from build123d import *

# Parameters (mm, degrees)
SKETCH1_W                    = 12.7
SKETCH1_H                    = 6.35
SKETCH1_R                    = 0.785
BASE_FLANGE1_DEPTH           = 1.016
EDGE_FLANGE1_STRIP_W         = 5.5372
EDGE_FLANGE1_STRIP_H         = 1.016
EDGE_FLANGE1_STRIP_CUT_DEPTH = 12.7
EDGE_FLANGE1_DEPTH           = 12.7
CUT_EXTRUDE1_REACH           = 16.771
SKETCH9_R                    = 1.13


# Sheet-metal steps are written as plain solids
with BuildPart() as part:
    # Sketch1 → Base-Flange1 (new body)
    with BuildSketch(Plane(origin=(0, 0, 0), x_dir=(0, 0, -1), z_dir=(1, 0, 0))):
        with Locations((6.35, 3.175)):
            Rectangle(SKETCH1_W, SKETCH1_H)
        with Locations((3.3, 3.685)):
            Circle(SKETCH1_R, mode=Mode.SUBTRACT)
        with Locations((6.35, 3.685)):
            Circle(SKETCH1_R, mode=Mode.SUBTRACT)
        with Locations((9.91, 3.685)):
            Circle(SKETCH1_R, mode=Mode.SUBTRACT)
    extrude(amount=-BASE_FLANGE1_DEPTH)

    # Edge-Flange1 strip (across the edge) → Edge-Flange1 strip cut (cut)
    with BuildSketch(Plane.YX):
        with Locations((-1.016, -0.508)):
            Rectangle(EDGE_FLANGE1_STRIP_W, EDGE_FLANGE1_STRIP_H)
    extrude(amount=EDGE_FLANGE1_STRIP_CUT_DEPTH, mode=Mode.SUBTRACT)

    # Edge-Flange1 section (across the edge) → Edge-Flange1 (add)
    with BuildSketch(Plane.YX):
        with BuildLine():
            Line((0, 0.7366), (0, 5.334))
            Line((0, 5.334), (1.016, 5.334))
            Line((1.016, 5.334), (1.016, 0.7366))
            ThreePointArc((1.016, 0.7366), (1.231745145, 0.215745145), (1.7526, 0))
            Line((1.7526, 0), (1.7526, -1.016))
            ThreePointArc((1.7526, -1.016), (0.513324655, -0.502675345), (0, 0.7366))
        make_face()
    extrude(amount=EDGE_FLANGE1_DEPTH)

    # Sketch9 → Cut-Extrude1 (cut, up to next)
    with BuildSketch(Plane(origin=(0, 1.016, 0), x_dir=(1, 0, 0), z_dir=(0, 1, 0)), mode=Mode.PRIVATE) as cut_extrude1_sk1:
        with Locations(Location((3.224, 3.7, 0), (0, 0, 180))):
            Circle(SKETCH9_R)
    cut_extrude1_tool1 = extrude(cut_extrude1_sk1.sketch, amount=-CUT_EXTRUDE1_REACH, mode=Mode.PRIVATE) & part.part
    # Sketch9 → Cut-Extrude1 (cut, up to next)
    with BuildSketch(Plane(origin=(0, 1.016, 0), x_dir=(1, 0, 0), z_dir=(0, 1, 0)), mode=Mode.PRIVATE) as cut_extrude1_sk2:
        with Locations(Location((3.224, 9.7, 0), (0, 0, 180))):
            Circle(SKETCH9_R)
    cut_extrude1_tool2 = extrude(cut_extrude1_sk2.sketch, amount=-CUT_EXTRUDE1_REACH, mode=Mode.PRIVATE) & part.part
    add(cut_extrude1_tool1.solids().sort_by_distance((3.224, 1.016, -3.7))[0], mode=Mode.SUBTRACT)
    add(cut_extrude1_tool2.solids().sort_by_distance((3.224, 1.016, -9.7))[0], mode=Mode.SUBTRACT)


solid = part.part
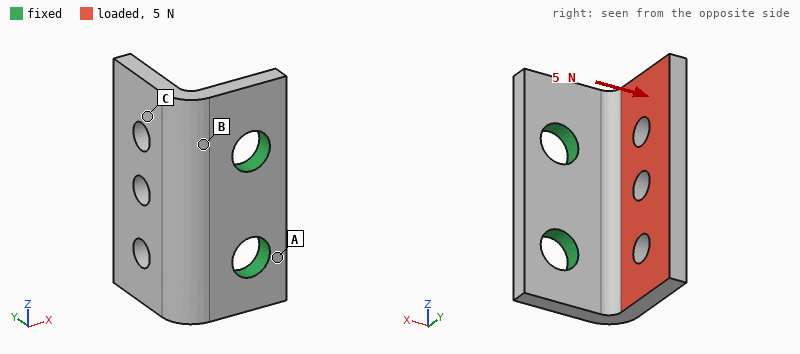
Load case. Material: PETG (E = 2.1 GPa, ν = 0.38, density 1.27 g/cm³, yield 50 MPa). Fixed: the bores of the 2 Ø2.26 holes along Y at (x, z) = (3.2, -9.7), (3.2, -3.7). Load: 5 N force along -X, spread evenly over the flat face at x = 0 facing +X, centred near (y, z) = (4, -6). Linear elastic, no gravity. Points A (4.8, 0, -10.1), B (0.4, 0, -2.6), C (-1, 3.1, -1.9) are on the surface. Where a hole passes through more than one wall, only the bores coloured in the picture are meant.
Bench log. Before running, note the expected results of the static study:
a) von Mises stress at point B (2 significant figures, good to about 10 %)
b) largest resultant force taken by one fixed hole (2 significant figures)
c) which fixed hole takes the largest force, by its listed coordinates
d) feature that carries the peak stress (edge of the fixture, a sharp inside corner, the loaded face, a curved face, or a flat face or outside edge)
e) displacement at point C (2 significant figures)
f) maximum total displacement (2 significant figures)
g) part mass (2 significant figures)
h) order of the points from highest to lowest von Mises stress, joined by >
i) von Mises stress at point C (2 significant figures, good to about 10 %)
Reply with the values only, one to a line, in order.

5.6 MPa
2.7 N
(3.2, -3.7)
a flat face or outside edge
0.082 mm
0.18 mm
0.16 g
B > C > A
3.4 MPa
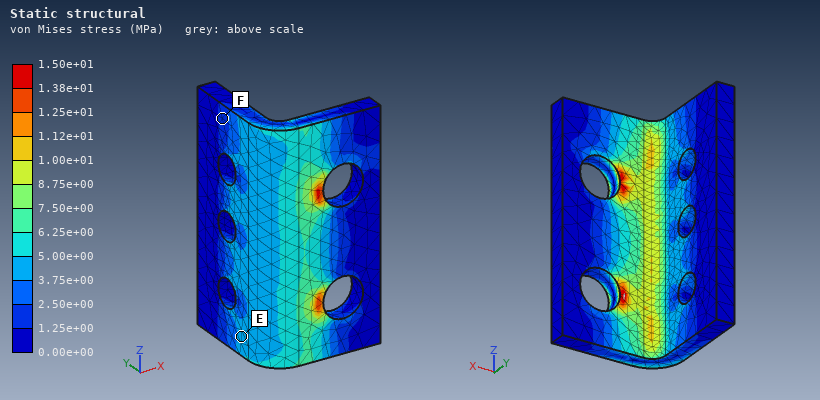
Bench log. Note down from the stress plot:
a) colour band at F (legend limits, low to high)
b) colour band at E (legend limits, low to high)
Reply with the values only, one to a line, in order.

1.25e+00 to 2.50e+00 MPa
3.75e+00 to 5.00e+00 MPa
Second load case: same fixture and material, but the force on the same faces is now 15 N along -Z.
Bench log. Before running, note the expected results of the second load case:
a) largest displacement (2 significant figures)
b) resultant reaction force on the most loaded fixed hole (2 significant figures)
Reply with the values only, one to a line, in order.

0.16 mm
12 N
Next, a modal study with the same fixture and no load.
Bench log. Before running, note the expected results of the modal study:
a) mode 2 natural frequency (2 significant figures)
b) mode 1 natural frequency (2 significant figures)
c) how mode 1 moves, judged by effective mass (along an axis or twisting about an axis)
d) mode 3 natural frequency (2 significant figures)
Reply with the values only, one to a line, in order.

5600 Hz
3700 Hz
along X
9600 Hz
